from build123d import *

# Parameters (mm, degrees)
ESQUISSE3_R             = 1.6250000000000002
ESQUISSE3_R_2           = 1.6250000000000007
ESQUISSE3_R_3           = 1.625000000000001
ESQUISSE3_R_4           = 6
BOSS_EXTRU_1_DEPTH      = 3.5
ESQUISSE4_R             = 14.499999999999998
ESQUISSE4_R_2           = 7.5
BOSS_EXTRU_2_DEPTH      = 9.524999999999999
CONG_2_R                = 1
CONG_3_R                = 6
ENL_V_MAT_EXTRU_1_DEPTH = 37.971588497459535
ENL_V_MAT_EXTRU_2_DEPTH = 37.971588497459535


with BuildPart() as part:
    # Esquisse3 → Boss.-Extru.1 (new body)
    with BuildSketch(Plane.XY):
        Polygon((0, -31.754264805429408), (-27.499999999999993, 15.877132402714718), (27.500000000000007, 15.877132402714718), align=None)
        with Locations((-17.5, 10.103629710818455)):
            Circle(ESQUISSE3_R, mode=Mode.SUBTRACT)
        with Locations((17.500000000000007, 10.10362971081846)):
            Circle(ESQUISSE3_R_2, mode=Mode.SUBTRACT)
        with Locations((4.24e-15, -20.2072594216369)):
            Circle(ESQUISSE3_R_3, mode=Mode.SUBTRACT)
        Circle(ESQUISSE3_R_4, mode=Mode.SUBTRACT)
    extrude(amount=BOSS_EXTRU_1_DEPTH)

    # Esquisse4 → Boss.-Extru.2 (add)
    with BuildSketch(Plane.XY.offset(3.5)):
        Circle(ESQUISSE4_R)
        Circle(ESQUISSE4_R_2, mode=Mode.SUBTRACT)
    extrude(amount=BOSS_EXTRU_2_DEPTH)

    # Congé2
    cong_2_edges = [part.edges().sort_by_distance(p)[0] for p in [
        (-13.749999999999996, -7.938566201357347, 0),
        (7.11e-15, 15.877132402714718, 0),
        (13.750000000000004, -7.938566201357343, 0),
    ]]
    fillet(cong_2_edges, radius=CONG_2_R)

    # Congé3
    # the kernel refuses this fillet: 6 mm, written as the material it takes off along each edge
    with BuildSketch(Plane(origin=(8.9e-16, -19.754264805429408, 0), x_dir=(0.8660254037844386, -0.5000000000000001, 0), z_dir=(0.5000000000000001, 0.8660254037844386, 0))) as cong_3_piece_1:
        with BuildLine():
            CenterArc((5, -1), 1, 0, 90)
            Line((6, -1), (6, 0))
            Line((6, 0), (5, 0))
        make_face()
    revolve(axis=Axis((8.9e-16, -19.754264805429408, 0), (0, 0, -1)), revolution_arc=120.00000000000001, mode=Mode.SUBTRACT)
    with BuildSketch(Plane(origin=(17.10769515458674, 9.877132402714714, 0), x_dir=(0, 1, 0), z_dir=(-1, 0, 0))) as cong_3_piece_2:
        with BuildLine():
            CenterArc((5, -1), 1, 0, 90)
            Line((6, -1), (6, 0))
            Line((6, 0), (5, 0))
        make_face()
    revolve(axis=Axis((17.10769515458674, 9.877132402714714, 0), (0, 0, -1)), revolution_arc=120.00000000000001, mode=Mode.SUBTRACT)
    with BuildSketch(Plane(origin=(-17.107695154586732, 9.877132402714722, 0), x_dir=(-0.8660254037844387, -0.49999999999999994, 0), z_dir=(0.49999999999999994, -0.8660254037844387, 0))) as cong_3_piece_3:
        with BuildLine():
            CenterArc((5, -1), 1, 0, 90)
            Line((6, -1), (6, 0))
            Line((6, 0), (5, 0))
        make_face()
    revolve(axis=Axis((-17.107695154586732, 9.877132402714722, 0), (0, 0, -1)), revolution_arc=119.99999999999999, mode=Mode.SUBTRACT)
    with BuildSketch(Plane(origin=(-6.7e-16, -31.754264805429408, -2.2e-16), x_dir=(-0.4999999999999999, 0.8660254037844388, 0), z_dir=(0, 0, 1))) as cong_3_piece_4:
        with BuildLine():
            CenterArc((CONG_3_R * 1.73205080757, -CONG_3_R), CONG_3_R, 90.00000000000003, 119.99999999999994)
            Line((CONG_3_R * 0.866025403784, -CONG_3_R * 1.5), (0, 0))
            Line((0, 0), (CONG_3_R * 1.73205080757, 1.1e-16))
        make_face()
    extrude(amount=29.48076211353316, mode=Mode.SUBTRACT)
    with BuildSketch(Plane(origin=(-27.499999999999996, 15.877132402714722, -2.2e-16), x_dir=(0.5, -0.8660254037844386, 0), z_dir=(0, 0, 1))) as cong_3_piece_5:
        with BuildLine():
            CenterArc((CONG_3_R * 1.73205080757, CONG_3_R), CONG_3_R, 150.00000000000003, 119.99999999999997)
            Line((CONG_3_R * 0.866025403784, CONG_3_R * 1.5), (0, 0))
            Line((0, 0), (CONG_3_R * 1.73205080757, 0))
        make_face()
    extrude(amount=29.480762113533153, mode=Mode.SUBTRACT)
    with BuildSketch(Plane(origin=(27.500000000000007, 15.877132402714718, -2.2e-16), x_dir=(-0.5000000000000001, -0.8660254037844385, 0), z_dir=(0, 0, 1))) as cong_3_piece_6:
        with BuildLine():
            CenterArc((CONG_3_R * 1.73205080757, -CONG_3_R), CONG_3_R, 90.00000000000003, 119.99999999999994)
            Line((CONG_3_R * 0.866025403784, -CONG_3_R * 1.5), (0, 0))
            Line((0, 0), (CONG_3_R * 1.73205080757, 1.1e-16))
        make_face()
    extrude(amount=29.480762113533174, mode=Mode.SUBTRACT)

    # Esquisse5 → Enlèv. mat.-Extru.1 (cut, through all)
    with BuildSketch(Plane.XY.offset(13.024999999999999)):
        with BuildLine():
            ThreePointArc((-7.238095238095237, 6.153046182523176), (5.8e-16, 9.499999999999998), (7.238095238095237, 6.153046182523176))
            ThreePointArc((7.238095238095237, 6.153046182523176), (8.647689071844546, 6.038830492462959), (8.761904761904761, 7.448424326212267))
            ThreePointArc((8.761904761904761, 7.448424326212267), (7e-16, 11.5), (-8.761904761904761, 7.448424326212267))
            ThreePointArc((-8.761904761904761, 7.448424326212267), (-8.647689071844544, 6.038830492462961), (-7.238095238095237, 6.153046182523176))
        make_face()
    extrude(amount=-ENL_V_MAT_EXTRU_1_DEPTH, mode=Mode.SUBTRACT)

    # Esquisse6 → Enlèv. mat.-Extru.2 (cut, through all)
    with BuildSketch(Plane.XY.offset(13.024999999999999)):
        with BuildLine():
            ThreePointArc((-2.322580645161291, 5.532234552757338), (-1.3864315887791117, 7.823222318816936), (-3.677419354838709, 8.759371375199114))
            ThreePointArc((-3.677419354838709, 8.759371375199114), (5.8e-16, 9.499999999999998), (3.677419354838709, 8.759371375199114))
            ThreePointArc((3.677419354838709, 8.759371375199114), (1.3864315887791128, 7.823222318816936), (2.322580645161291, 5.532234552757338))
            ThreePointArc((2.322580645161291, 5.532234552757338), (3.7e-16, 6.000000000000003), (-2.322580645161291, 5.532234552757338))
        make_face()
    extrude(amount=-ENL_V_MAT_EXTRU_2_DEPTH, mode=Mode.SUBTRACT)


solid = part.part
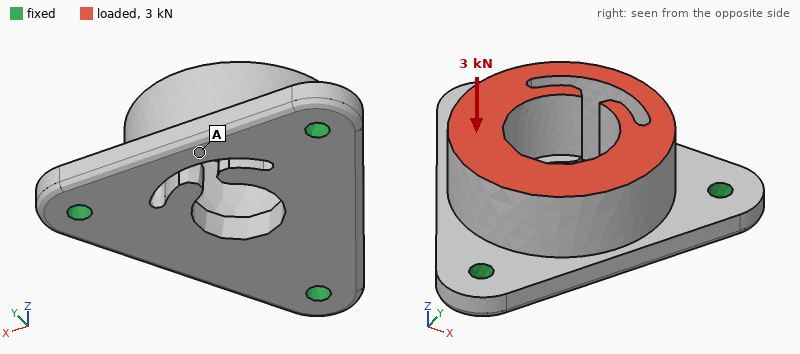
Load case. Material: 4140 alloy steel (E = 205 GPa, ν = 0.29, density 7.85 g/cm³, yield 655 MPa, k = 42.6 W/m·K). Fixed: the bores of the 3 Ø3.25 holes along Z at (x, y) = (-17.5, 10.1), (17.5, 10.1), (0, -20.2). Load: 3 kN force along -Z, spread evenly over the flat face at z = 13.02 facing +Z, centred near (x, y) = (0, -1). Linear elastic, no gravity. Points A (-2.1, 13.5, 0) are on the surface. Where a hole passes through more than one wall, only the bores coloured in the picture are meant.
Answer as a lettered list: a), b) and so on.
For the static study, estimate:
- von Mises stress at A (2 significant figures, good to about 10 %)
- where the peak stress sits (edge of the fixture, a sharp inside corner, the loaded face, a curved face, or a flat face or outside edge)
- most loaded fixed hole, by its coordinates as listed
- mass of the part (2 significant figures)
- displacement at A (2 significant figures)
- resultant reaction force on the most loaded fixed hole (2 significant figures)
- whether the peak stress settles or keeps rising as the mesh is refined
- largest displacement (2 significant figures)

a) 24 MPa
b) edge of the fixture
c) (0, -20.2)
d) 61 g
e) 7.4 µm
f) 1.2 kN
g) keeps rising
h) 8.9 µm
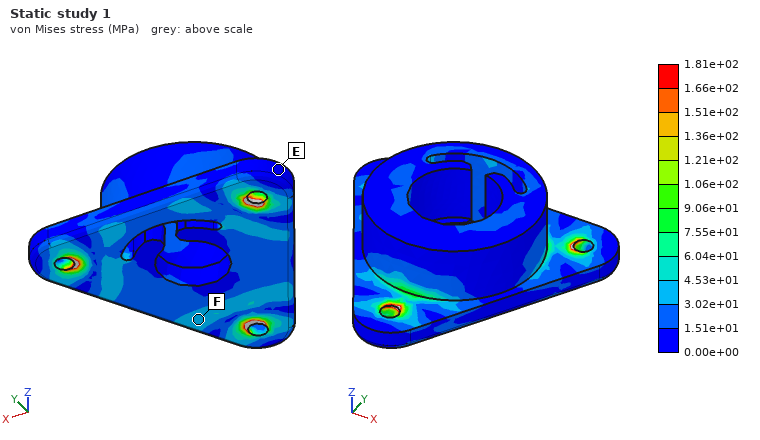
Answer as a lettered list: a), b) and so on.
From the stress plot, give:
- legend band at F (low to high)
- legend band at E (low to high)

a) 3.02e+01 to 4.53e+01 MPa
b) 0.00e+00 to 1.51e+01 MPa
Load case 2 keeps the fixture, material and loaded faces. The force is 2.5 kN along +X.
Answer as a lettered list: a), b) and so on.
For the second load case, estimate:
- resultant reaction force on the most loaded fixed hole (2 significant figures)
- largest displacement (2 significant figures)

a) 1.3 kN
b) 14 µm
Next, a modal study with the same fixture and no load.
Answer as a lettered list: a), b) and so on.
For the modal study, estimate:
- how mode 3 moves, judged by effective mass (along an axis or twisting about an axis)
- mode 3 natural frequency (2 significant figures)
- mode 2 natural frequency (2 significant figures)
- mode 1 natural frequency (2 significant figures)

a) along Y
b) 16 kHz
c) 15 kHz
d) 14 kHz
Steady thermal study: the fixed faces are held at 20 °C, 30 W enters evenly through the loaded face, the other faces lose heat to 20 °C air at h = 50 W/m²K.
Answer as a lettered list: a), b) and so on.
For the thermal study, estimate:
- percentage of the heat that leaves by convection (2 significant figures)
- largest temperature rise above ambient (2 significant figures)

a) 19 %
b) 49 K
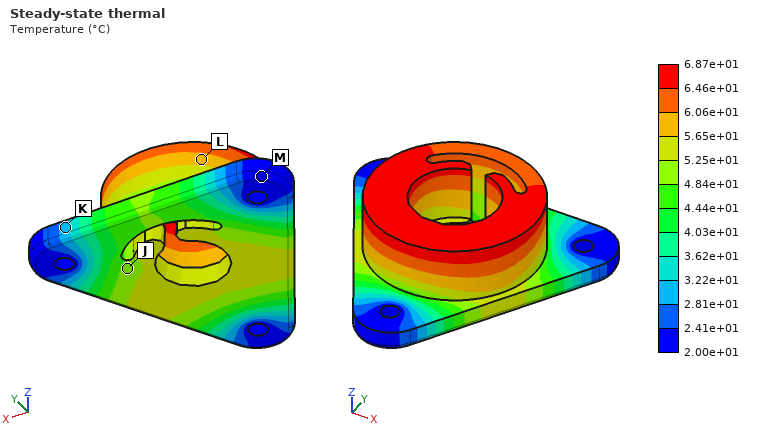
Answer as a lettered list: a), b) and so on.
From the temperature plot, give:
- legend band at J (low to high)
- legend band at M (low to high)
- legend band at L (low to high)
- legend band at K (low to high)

a) 4.84e+01 to 5.25e+01 °C
b) 2.00e+01 to 2.41e+01 °C
c) 5.65e+01 to 6.06e+01 °C
d) 2.81e+01 to 3.22e+01 °C
